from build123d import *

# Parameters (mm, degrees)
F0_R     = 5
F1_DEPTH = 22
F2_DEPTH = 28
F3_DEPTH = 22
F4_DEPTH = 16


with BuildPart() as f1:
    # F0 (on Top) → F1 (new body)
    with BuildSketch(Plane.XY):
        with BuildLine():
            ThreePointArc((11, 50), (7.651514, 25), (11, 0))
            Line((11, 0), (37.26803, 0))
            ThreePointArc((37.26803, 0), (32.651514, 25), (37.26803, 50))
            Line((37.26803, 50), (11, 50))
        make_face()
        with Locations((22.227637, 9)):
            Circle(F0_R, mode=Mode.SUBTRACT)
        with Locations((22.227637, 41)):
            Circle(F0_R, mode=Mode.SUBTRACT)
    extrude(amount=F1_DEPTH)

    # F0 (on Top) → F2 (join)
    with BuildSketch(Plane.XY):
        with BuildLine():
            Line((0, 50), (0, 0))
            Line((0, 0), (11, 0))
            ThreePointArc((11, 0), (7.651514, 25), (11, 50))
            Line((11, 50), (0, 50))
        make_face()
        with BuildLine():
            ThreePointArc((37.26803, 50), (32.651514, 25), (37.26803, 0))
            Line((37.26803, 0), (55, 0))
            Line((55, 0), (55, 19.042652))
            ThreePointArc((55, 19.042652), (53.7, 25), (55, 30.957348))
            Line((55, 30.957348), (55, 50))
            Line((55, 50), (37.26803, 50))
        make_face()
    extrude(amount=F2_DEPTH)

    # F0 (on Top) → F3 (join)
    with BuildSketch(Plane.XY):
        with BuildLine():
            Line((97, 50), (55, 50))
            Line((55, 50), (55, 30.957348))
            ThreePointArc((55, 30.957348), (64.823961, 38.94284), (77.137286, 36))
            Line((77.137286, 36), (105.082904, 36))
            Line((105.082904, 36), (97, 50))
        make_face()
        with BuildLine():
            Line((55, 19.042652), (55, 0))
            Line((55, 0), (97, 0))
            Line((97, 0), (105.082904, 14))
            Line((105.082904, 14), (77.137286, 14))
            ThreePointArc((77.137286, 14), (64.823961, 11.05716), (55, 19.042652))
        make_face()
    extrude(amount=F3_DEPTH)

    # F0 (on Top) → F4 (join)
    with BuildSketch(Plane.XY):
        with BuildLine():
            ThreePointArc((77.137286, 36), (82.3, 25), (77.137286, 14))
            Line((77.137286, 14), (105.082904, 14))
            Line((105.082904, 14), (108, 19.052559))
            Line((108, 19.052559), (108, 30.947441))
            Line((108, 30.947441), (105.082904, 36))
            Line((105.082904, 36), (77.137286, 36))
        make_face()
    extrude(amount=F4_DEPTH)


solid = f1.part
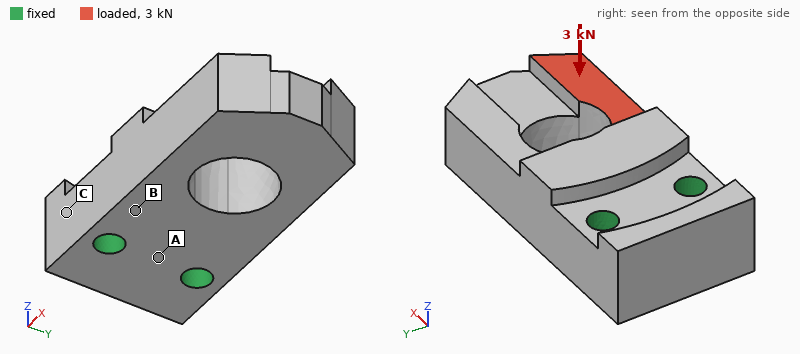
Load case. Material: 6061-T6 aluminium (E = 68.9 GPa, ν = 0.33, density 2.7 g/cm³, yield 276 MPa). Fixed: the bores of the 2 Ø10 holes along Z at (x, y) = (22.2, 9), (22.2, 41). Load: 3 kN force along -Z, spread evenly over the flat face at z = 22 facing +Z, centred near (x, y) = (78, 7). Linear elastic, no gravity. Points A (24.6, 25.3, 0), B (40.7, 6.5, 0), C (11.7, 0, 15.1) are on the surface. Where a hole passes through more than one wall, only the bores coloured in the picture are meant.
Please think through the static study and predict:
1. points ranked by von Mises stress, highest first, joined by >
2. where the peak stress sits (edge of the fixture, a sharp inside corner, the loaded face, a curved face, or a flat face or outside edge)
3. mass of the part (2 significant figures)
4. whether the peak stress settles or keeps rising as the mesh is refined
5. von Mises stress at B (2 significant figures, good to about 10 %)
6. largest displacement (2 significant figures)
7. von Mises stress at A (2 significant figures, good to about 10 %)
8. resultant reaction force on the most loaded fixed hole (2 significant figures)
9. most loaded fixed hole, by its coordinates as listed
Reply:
B > A > C
edge of the fixture
280 g
keeps rising
36 MPa
0.13 mm
17 MPa
2.7 kN
(22.2, 9)
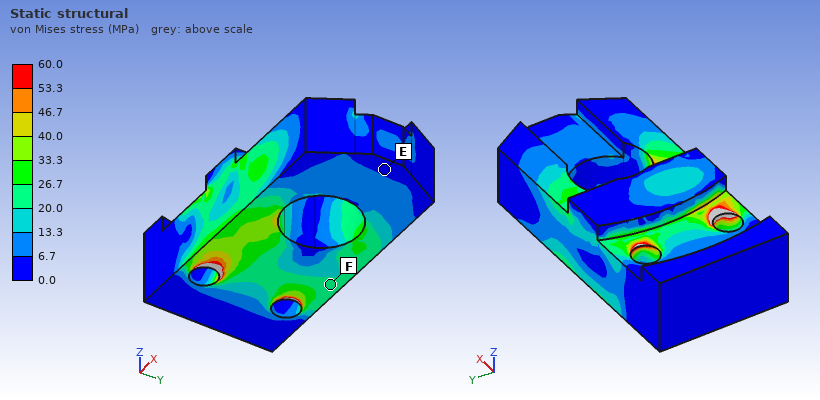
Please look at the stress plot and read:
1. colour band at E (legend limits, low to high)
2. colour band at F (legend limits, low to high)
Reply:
0.0 to 6.7 MPa
20.0 to 26.7 MPa
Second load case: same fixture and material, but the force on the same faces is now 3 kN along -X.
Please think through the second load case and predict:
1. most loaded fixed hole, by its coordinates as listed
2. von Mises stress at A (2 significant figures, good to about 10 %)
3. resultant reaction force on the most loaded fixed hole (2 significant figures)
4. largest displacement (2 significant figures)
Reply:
(22.2, 9)
2.8 MPa
3.0 kN
48 µm
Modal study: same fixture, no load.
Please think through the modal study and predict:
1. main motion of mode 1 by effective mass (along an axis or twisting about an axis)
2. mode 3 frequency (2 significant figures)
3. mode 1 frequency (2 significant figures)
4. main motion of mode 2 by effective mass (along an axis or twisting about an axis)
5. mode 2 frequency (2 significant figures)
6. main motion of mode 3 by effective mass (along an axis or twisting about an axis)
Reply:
along Z
6800 Hz
2800 Hz
along Y
4600 Hz
twisting about X
